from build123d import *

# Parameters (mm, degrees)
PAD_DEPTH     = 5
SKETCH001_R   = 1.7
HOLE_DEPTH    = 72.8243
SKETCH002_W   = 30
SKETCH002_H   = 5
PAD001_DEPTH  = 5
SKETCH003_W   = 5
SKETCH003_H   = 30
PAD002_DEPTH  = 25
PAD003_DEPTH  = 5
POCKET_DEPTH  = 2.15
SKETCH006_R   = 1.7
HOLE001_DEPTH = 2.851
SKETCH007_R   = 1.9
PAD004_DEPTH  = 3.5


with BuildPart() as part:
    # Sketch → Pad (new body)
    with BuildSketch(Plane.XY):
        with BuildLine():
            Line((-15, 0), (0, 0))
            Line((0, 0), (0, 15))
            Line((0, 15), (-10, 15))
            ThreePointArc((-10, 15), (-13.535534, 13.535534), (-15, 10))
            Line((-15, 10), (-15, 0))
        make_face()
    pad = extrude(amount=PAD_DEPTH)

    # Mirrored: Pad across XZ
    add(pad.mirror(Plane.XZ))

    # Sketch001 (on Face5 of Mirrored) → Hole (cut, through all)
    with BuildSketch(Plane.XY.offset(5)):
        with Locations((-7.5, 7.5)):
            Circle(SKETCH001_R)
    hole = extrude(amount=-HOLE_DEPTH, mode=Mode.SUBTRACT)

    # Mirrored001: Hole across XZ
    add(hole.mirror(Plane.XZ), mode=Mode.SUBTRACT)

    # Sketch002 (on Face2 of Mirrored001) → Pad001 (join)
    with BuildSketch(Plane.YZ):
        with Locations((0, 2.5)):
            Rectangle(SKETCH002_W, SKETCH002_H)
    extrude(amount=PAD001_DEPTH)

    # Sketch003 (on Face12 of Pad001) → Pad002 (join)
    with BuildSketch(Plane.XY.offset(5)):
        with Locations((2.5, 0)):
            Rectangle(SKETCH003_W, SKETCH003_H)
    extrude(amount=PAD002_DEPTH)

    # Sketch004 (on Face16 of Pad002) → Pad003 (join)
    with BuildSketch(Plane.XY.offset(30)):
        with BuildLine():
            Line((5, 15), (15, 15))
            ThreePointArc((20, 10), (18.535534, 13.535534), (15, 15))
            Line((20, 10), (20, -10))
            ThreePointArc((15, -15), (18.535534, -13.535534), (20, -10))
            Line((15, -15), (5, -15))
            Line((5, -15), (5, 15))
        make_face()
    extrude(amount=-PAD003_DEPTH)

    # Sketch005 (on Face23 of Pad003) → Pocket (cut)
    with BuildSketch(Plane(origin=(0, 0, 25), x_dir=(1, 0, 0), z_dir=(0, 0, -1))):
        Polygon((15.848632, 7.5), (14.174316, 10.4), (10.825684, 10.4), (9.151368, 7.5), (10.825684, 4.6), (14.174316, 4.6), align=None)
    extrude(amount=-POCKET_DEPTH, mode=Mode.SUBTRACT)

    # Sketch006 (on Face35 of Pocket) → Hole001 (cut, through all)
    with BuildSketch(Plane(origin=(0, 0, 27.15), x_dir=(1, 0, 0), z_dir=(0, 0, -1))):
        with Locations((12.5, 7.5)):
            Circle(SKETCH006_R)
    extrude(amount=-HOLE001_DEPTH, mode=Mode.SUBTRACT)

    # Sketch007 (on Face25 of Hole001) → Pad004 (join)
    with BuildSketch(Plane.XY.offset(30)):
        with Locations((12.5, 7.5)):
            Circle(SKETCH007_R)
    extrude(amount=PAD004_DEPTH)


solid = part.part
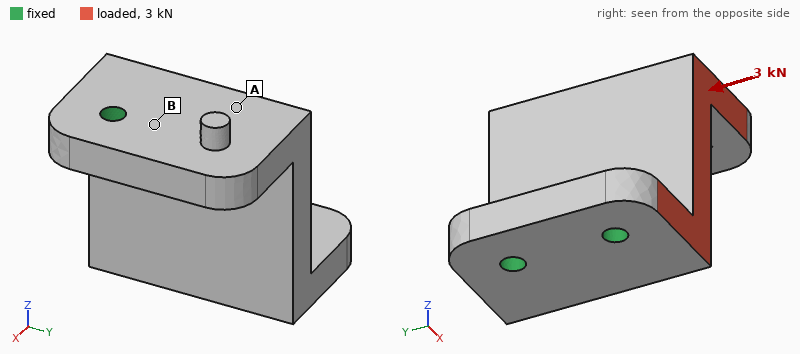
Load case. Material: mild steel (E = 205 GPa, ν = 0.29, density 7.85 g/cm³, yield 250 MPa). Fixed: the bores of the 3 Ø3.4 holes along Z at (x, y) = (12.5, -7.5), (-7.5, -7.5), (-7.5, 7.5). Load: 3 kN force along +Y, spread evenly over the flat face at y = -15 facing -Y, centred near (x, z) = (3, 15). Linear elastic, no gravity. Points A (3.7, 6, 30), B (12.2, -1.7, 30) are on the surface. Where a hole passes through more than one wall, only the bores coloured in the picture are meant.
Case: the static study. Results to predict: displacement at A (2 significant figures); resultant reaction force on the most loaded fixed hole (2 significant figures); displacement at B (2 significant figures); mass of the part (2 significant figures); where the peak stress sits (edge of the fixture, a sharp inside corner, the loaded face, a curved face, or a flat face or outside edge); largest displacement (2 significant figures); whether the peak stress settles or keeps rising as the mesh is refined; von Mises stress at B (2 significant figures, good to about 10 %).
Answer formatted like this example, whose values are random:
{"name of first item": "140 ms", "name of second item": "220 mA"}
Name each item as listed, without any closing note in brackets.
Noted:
{"displacement at A": "9.8 µm", "resultant reaction force on the most loaded fixed hole": "1.3 kN", "displacement at B": "3.2 µm", "mass of the part": "69 g", "where the peak stress sits": "edge of the fixture", "largest displacement": "15 µm", "whether the peak stress settles or keeps rising as the mesh is refined": "keeps rising", "von Mises stress at B": "25 MPa"}
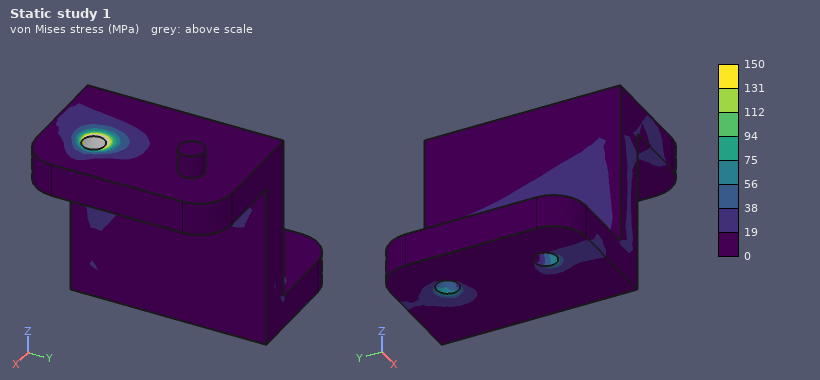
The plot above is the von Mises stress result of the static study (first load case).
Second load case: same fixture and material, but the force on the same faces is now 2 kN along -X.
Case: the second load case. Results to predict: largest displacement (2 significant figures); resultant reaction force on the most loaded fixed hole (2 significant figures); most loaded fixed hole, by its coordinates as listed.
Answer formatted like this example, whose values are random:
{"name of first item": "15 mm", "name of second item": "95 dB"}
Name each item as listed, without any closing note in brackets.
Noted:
{"largest displacement": "14 µm", "resultant reaction force on the most loaded fixed hole": "1.4 kN", "most loaded fixed hole, by its coordinates as listed": "(-7.5, -7.5)"}
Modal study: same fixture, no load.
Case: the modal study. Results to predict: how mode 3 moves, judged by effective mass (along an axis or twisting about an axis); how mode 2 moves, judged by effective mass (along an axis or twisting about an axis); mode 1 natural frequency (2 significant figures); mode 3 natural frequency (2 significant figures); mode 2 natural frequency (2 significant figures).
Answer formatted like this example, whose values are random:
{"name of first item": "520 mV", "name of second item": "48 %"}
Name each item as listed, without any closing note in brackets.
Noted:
{"how mode 3 moves, judged by effective mass": "along Z", "how mode 2 moves, judged by effective mass": "along Z", "mode 1 natural frequency": "7900 Hz", "mode 3 natural frequency": "15 kHz", "mode 2 natural frequency": "13 kHz"}
